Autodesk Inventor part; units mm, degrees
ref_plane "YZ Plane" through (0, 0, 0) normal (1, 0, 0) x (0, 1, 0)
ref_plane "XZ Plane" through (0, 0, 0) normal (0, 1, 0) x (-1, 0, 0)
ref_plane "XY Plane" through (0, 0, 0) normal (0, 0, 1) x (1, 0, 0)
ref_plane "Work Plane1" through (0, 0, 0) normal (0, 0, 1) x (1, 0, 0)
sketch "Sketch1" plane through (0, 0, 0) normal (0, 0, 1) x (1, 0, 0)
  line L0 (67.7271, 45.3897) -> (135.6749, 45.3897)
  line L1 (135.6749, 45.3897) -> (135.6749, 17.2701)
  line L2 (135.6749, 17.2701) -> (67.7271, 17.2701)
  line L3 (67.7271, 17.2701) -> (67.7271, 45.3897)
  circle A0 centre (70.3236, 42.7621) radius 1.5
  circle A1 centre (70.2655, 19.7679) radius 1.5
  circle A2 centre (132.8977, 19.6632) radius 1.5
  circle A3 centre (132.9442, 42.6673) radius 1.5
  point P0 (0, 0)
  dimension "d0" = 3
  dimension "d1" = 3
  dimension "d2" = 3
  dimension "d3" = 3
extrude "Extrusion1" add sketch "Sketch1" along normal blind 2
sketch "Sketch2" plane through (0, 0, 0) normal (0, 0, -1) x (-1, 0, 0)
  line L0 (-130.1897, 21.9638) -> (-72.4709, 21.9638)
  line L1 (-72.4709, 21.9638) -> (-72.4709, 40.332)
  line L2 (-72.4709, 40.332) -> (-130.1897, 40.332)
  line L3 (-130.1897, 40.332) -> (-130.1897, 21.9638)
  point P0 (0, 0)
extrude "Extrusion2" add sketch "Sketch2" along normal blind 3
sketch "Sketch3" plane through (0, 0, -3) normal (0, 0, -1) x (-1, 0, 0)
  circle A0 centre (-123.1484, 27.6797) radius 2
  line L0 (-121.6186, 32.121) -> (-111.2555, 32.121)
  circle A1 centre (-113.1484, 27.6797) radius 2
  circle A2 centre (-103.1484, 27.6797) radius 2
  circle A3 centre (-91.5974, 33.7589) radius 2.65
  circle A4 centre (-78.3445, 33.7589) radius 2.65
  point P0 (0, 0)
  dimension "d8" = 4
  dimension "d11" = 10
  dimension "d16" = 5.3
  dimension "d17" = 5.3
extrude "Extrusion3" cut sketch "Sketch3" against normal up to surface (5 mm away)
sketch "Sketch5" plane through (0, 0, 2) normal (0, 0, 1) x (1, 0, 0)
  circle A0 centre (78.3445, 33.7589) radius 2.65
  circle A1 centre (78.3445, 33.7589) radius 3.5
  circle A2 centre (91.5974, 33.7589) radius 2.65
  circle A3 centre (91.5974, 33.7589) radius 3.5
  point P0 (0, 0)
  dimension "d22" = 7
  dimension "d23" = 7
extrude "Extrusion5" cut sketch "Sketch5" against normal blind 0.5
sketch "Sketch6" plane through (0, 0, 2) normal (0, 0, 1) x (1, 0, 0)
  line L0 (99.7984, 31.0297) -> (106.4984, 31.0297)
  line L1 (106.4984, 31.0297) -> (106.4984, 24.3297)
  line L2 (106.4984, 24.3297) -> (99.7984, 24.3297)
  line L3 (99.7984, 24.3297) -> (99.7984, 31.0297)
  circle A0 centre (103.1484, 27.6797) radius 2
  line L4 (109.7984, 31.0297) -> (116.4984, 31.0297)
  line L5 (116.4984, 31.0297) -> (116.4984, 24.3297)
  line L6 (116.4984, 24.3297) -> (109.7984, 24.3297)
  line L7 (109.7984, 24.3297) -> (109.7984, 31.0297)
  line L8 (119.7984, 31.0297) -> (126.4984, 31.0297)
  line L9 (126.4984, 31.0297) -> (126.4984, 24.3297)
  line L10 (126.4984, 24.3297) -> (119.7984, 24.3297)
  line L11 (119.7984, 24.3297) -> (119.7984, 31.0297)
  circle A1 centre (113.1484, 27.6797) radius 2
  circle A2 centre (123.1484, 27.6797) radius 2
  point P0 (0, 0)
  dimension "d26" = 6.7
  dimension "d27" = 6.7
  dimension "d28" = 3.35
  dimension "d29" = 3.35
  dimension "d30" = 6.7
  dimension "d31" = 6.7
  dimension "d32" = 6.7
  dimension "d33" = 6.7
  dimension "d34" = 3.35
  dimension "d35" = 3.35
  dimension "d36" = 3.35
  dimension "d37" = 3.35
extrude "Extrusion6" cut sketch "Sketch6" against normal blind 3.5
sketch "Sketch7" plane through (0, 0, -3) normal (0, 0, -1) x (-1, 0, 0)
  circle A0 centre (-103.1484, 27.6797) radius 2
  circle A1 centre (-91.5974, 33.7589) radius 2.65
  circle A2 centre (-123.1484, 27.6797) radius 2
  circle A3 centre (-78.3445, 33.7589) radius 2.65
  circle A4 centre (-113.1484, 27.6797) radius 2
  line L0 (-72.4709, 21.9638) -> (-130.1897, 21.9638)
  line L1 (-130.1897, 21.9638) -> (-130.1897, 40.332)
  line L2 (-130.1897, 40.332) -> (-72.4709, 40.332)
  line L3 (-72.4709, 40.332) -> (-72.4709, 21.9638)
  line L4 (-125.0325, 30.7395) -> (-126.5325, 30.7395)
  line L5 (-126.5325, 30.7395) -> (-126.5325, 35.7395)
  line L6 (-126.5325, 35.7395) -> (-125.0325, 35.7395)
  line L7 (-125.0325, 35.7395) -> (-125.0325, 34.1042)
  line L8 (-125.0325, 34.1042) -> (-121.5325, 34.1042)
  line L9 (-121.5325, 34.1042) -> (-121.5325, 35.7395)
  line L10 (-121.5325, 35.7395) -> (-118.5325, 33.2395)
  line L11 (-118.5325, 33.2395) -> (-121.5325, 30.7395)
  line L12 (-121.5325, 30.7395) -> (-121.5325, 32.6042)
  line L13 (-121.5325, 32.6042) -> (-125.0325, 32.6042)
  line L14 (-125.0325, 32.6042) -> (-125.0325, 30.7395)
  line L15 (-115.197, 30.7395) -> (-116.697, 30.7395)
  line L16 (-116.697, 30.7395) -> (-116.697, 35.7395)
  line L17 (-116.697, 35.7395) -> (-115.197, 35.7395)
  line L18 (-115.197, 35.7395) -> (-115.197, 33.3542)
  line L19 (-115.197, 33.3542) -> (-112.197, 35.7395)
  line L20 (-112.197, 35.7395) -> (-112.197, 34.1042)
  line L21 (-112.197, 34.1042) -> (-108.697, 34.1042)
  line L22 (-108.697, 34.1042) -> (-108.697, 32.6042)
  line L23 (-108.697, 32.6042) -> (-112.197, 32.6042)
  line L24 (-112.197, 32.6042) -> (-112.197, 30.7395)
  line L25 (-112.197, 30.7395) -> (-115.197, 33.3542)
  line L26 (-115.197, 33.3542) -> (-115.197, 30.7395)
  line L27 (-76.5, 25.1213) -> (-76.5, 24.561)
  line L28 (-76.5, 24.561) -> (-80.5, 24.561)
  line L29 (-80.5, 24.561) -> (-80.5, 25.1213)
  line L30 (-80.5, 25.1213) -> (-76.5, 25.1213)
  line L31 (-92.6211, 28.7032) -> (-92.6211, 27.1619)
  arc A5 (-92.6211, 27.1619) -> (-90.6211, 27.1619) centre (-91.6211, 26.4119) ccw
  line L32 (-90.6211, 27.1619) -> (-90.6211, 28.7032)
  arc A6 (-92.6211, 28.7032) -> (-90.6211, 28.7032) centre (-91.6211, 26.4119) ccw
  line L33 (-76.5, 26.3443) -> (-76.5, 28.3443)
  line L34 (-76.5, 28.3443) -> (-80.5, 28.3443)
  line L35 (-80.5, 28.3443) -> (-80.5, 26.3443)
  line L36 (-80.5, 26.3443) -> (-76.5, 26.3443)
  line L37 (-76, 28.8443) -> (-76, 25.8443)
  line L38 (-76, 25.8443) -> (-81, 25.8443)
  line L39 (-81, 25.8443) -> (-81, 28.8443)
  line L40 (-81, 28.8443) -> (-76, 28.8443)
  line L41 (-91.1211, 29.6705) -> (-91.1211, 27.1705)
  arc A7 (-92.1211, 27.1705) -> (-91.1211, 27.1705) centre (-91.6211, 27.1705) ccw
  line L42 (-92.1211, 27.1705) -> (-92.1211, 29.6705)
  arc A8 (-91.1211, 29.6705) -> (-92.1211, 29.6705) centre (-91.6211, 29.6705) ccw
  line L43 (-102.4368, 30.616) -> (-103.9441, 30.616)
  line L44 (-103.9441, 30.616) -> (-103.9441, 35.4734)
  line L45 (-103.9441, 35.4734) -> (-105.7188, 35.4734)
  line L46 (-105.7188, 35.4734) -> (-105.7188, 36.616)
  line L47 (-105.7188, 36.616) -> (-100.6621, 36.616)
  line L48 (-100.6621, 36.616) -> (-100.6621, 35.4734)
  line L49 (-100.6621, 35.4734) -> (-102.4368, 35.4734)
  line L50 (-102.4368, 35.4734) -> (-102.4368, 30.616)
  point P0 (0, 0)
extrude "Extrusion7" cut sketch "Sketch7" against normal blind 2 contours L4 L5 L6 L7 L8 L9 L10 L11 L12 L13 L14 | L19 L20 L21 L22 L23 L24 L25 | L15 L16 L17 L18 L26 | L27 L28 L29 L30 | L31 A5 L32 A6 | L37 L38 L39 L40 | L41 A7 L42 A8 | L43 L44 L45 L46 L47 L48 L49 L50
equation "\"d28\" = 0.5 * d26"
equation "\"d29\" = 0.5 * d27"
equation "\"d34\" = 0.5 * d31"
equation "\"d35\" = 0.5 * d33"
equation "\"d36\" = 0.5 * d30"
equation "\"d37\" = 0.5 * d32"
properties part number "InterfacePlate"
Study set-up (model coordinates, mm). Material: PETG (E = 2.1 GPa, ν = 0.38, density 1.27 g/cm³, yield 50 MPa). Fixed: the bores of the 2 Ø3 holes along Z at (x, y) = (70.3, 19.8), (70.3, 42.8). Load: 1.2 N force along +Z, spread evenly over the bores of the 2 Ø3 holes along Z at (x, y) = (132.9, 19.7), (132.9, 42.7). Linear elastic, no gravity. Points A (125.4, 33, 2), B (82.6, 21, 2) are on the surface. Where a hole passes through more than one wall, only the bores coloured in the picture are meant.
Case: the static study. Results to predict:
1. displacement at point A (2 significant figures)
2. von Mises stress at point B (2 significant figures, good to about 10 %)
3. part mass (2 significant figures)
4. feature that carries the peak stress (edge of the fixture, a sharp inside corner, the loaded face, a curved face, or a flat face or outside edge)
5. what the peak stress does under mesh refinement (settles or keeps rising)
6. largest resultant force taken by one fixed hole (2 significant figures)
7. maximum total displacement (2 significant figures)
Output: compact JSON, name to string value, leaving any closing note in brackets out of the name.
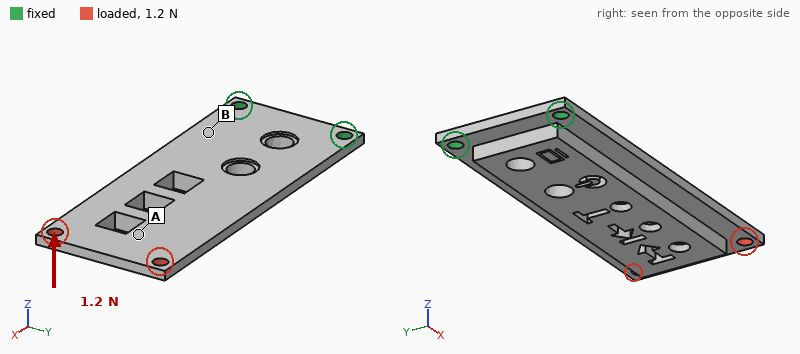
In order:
{"displacement at point A": "0.65 mm", "von Mises stress at point B": "0.82 MPa", "part mass": "7.7 g", "feature that carries the peak stress": "edge of the fixture", "what the peak stress does under mesh refinement": "keeps rising", "largest resultant force taken by one fixed hole": "0.62 N", "maximum total displacement": "0.81 mm"}
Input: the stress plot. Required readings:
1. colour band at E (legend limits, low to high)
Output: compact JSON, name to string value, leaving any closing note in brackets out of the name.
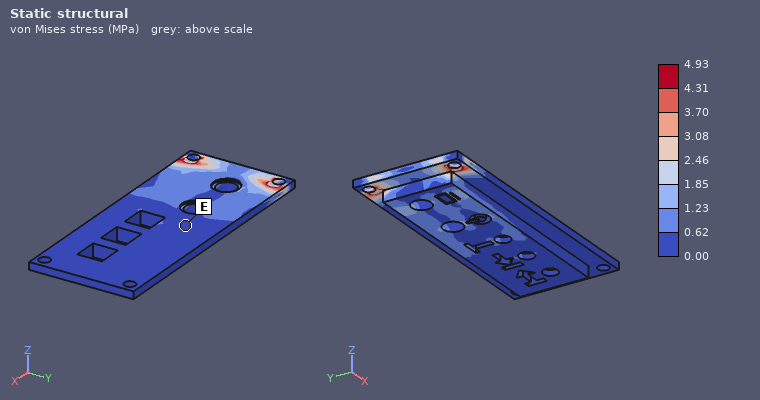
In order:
{"colour band at E": "0.00 to 0.62 MPa"}
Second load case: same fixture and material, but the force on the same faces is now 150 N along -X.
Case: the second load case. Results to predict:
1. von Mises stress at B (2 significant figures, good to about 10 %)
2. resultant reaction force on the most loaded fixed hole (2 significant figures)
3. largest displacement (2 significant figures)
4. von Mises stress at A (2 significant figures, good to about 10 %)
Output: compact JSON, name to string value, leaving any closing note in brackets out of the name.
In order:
{"von Mises stress at B": "3.9 MPa", "resultant reaction force on the most loaded fixed hole": "78 N", "largest displacement": "0.87 mm", "von Mises stress at A": "2.3 MPa"}
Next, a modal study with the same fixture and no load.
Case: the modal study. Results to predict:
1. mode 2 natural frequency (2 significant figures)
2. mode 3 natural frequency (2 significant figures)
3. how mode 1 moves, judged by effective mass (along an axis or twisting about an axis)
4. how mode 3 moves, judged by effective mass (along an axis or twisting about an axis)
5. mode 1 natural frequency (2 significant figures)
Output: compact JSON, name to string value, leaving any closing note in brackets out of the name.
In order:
{"mode 2 natural frequency": "890 Hz", "mode 3 natural frequency": "1100 Hz", "how mode 1 moves, judged by effective mass": "along Z", "how mode 3 moves, judged by effective mass": "along Z", "mode 1 natural frequency": "130 Hz"}
